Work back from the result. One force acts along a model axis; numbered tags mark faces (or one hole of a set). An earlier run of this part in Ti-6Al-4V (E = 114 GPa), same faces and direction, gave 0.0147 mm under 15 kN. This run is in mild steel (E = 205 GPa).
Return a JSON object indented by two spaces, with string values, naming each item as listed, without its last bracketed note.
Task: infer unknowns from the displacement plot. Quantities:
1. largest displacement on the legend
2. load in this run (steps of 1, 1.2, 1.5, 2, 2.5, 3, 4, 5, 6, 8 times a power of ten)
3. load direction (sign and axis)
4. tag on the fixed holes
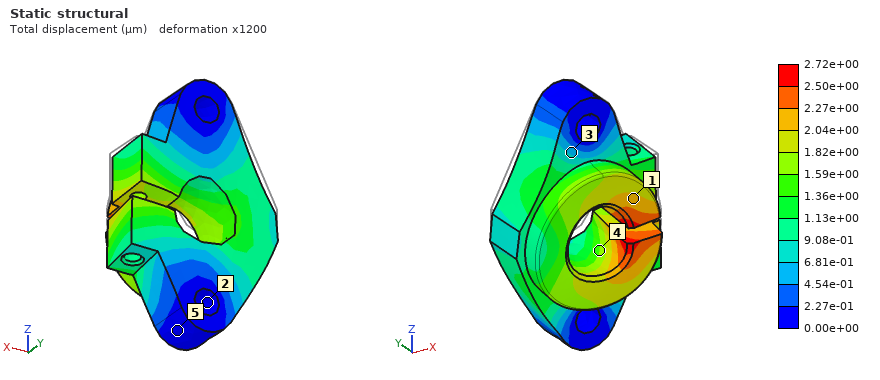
{
  "largest displacement on the legend": "2.72e+00 µm",
  "load in this run": "5 kN",
  "load direction": "-Z",
  "tag on the fixed holes": "2"
}
